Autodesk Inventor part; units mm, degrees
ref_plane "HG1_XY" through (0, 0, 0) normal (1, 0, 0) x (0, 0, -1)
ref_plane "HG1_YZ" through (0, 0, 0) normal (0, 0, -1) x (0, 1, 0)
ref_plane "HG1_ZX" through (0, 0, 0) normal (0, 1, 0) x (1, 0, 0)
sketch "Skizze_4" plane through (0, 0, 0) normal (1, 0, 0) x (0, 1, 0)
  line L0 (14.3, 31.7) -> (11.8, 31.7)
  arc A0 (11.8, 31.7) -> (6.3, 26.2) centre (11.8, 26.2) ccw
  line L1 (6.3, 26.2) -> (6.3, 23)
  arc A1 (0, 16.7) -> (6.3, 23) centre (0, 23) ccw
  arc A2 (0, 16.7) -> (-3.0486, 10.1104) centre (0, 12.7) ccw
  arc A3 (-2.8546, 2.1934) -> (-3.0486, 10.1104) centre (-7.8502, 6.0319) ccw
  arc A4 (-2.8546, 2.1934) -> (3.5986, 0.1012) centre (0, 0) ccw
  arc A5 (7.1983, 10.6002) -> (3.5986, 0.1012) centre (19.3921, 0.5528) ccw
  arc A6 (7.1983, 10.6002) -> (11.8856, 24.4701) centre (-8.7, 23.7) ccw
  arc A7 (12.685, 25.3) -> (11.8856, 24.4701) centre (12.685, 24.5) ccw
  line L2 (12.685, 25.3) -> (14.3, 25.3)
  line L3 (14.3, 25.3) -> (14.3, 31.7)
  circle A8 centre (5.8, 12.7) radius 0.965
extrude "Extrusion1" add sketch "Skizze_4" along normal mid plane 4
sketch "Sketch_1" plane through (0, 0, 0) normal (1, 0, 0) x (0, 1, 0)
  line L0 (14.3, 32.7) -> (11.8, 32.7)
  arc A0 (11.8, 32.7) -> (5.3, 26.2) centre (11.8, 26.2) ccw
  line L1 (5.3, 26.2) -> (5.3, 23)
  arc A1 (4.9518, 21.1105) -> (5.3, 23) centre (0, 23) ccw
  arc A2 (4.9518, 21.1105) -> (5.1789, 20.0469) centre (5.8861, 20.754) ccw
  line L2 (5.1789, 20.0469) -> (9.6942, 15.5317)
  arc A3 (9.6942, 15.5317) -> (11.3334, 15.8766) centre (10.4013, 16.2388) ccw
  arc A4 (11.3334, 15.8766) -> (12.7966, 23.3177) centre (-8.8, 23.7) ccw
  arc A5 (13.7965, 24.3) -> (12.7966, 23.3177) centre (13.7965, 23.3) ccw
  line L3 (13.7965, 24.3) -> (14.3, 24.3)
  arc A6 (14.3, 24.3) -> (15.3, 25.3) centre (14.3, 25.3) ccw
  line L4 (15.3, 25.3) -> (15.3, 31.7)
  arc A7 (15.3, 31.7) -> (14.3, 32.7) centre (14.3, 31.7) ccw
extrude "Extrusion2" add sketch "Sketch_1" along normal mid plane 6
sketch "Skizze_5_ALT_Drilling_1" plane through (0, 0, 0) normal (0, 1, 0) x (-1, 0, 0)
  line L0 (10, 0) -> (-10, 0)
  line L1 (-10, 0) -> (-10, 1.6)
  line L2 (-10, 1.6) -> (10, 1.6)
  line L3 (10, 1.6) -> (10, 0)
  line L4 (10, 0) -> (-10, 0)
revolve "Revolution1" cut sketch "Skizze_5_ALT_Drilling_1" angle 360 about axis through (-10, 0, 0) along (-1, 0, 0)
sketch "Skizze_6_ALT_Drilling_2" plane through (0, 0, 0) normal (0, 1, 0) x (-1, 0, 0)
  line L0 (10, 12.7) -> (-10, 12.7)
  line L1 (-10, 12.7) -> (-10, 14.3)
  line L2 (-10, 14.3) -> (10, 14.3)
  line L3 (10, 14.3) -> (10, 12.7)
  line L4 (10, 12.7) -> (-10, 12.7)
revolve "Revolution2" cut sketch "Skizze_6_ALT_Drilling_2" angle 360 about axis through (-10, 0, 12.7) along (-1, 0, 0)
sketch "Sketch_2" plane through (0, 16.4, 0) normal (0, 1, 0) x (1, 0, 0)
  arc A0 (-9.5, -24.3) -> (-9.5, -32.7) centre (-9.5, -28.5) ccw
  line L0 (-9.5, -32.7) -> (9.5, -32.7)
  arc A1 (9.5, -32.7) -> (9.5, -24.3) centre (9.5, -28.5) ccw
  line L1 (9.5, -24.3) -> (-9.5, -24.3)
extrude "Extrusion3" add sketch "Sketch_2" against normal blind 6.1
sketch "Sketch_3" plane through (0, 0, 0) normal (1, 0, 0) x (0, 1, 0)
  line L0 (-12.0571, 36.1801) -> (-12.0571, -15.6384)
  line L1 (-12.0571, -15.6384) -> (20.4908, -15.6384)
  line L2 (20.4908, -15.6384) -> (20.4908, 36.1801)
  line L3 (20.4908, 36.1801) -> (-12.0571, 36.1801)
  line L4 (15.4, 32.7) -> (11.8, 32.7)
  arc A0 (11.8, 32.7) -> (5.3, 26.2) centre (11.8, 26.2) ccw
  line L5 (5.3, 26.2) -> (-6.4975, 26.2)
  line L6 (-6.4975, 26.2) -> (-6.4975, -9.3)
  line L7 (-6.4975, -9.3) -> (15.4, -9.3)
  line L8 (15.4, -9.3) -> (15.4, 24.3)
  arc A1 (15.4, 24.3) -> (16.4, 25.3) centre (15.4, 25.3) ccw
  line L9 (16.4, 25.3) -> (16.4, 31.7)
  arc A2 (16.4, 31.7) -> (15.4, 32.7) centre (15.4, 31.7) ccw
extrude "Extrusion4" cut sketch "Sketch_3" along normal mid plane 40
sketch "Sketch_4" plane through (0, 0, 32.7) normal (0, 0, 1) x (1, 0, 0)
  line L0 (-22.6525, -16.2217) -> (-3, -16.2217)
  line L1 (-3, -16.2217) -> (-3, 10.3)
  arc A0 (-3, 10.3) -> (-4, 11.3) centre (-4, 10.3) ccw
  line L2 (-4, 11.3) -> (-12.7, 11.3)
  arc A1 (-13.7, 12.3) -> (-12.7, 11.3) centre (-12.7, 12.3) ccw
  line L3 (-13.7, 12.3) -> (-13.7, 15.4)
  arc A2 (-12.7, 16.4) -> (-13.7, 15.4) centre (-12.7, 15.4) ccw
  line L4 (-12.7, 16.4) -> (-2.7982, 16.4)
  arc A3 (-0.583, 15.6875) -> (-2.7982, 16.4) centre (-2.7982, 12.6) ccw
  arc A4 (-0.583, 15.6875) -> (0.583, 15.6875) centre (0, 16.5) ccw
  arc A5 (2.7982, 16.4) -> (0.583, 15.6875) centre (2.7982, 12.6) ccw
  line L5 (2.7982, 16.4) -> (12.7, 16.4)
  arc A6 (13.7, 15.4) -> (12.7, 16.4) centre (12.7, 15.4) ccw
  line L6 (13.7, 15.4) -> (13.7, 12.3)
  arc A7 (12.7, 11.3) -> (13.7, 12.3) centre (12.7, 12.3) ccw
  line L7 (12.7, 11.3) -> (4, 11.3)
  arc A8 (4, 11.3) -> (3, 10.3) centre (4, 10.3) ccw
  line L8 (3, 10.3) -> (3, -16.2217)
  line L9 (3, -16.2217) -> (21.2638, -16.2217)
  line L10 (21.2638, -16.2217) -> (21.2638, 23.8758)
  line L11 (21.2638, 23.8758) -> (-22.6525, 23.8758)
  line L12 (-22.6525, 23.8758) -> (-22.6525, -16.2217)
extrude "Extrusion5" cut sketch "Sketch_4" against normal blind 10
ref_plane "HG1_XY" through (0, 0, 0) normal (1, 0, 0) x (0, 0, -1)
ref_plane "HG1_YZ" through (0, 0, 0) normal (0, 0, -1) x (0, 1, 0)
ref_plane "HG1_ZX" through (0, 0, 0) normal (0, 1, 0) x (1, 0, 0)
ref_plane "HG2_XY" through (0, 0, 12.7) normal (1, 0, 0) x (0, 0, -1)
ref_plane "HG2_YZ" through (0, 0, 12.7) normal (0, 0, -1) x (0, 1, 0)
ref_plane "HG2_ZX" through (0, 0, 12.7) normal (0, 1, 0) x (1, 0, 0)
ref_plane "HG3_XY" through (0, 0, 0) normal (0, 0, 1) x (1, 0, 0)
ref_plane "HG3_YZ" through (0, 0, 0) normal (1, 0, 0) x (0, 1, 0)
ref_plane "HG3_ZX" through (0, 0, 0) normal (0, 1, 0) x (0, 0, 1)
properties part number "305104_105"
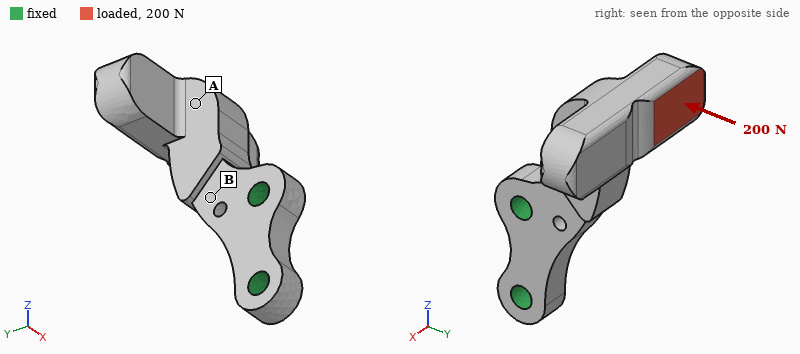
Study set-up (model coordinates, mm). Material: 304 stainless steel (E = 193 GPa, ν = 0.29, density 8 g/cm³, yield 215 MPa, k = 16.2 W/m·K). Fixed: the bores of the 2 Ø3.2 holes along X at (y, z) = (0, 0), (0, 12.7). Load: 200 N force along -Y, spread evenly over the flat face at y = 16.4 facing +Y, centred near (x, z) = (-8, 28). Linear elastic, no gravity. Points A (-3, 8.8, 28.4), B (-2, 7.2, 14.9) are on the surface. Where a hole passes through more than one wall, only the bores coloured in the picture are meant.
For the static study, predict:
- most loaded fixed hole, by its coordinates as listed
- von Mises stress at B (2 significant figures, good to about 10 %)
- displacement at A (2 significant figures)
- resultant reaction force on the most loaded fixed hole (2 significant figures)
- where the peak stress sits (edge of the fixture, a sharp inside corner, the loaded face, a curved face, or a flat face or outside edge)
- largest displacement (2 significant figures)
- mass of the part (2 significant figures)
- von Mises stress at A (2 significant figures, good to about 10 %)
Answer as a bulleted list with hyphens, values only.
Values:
- (0, 12.7)
- 68 MPa
- 26 µm
- 410 N
- a curved face
- 65 µm
- 18 g
- 24 MPa
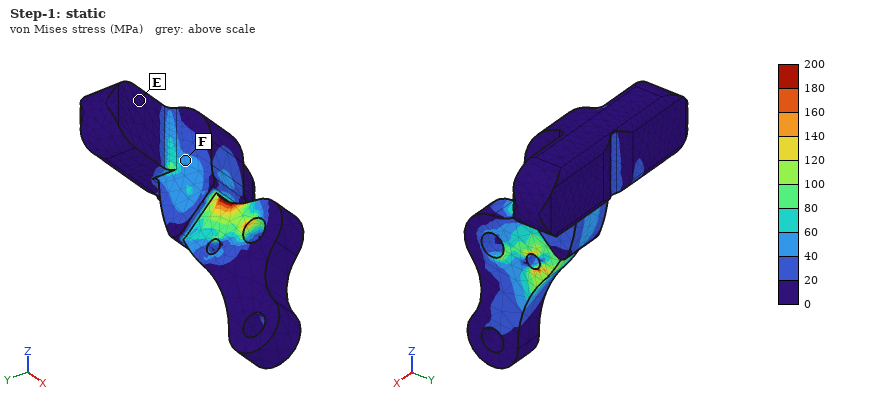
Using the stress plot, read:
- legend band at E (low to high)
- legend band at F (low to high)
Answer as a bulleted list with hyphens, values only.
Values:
- 0 to 20 MPa
- 40 to 60 MPa
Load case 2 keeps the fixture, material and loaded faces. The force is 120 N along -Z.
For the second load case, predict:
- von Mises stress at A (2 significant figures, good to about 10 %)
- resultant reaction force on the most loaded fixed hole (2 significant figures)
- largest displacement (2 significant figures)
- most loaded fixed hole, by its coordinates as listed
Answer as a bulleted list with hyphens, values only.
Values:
- 8.1 MPa
- 160 N
- 36 µm
- (0, 0)
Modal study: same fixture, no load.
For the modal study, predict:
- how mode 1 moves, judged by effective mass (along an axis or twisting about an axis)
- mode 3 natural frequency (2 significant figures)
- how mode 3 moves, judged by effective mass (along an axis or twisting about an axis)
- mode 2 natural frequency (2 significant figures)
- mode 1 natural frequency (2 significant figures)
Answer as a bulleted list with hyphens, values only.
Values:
- along X
- 5300 Hz
- twisting about Z
- 4400 Hz
- 2400 Hz
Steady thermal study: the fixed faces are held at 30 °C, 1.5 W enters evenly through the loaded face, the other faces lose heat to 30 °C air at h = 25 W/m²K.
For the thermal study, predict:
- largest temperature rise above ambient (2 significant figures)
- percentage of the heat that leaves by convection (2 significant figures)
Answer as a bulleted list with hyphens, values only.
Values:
- 43 K
- 47 %
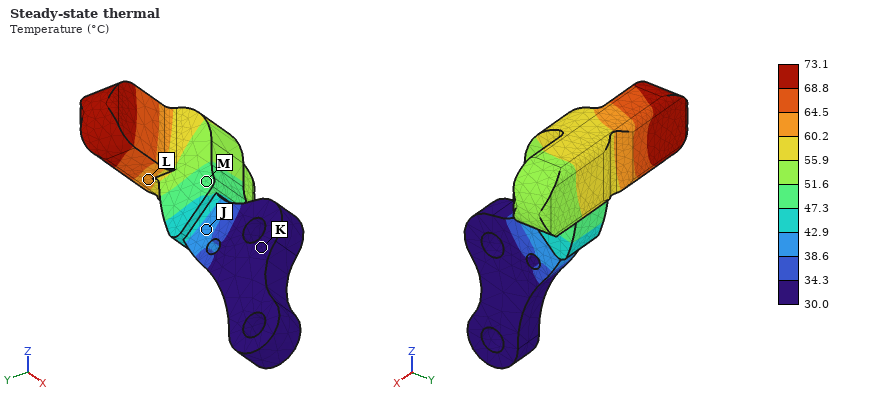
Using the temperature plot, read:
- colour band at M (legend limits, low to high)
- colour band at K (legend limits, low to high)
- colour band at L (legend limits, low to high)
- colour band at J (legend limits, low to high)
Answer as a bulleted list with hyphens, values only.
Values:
- 47.3 to 51.6 °C
- 30.0 to 34.3 °C
- 60.2 to 64.5 °C
- 38.6 to 42.9 °C
